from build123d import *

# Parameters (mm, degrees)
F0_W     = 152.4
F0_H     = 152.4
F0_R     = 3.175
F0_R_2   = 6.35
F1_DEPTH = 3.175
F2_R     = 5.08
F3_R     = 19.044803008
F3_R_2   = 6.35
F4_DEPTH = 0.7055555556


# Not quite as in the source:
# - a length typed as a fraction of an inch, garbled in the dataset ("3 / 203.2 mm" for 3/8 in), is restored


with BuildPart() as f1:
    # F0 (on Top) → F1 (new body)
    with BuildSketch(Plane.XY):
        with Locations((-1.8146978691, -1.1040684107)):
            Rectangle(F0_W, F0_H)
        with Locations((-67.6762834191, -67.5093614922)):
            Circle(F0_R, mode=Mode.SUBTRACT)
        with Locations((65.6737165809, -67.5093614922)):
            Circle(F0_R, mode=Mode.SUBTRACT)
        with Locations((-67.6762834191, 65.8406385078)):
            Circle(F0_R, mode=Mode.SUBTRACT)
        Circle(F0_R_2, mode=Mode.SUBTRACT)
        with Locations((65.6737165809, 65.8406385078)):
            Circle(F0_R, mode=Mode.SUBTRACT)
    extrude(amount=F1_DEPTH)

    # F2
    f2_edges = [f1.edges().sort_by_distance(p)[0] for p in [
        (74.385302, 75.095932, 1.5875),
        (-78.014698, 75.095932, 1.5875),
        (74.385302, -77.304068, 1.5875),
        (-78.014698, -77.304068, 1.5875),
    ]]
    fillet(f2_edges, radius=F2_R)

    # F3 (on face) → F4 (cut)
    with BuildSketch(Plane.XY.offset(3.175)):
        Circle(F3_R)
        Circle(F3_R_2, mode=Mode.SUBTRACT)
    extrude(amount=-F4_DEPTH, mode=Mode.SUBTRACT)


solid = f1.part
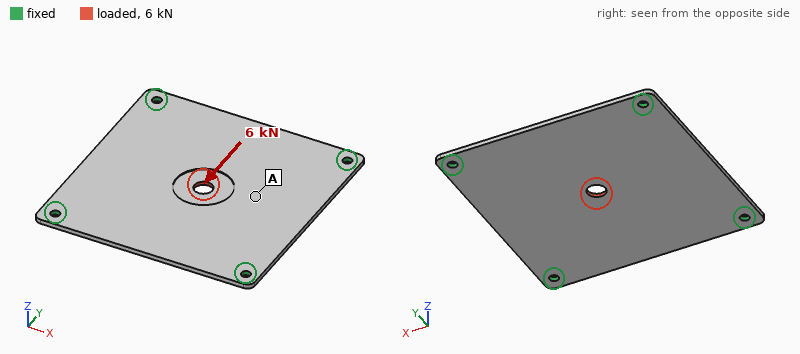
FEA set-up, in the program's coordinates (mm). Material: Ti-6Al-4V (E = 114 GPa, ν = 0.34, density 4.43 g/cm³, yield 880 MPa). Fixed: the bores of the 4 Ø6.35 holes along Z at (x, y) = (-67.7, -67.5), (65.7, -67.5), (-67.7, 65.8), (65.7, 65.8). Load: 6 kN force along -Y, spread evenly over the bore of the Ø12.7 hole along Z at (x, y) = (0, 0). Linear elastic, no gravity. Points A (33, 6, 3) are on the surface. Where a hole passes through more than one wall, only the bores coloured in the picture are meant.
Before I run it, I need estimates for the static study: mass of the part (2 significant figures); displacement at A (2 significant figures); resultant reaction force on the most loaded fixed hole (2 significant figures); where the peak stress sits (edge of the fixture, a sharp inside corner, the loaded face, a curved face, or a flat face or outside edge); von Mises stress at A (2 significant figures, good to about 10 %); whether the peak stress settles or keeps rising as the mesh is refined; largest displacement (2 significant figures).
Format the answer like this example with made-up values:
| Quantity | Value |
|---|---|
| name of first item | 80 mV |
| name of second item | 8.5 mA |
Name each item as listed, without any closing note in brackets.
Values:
| Quantity | Value |
|---|---|
| mass of the part | 320 g |
| displacement at A | 9.3 µm |
| resultant reaction force on the most loaded fixed hole | 1.7 kN |
| where the peak stress sits | a sharp inside corner |
| von Mises stress at A | 9.7 MPa |
| whether the peak stress settles or keeps rising as the mesh is refined | keeps rising |
| largest displacement | 21 µm |
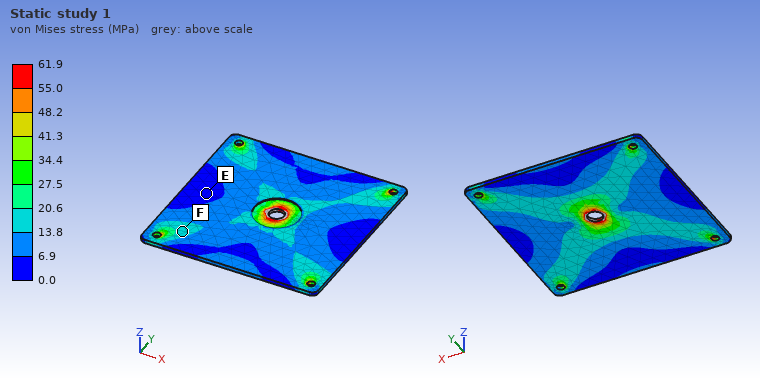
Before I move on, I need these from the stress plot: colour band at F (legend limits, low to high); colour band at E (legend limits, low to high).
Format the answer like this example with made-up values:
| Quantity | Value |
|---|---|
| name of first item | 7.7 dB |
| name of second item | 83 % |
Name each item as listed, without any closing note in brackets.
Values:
| Quantity | Value |
|---|---|
| colour band at F | 13.8 to 20.6 MPa |
| colour band at E | 0.0 to 6.9 MPa |
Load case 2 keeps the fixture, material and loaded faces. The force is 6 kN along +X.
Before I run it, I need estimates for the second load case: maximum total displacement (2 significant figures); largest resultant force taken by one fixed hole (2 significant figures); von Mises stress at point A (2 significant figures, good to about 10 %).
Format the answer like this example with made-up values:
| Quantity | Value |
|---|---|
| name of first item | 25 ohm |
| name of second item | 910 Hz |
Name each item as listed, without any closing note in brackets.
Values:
| Quantity | Value |
|---|---|
| maximum total displacement | 21 µm |
| largest resultant force taken by one fixed hole | 1.7 kN |
| von Mises stress at point A | 10 MPa |
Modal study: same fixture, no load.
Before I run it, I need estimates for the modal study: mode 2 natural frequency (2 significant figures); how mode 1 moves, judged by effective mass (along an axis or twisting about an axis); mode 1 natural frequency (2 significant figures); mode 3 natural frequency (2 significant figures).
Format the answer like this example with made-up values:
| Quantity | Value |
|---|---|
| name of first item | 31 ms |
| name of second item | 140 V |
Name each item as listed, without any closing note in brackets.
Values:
| Quantity | Value |
|---|---|
| mode 2 natural frequency | 1100 Hz |
| how mode 1 moves, judged by effective mass | along Z |
| mode 1 natural frequency | 600 Hz |
| mode 3 natural frequency | 1100 Hz |
